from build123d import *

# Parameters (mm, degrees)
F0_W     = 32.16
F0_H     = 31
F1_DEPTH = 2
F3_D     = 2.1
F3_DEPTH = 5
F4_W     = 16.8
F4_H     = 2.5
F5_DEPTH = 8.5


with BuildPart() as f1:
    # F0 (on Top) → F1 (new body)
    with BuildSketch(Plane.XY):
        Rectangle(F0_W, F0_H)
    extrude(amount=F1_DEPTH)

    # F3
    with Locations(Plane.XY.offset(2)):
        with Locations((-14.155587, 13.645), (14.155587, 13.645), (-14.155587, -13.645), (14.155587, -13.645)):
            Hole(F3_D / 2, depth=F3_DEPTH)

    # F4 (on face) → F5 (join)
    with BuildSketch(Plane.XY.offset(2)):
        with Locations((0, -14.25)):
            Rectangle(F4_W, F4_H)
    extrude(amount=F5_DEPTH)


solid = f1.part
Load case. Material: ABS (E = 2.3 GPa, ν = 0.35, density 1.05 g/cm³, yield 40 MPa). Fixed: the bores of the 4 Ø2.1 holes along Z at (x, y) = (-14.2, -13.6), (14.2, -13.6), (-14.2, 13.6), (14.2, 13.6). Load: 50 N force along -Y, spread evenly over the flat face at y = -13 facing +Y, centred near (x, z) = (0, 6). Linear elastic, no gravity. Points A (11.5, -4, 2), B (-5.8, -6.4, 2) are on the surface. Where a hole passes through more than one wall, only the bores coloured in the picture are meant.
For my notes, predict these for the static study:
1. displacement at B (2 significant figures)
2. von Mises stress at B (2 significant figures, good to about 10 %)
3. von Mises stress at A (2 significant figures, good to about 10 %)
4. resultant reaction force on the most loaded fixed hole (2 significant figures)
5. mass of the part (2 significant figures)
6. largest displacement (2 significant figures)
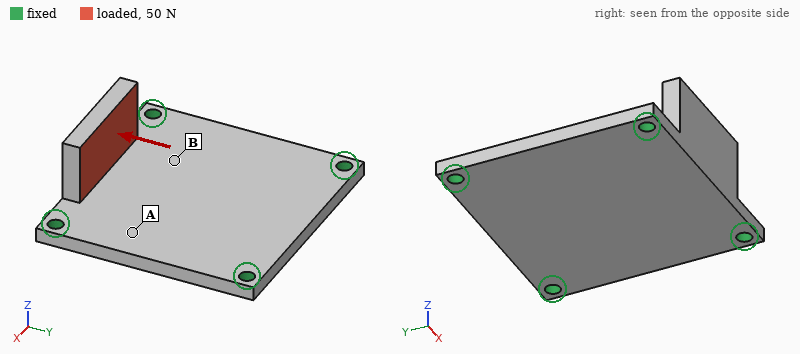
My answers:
0.089 mm
6.0 MPa
2.9 MPa
17 N
2.4 g
0.47 mm
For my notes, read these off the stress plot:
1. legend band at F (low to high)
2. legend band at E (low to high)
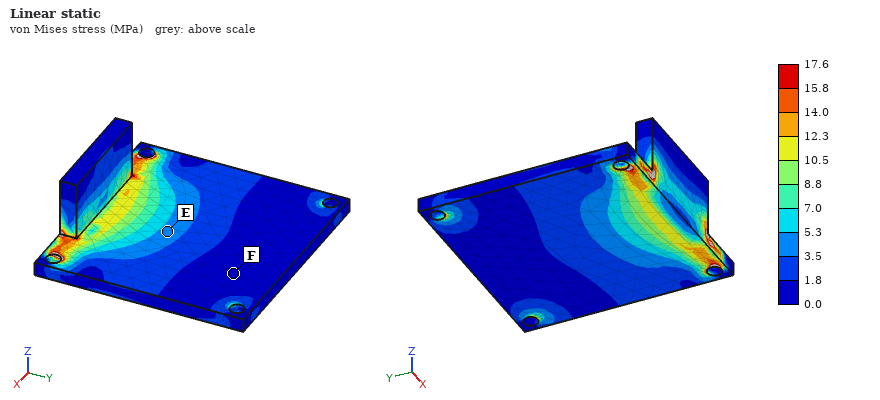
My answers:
0.0 to 1.8 MPa
3.5 to 5.3 MPa
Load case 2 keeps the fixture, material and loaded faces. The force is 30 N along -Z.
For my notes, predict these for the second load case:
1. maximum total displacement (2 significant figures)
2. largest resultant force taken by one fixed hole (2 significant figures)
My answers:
62 µm
16 N
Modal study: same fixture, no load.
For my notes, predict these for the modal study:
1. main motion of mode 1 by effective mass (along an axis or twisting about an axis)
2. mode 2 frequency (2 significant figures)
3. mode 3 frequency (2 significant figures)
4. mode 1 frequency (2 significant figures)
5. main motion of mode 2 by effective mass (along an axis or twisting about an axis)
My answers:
along Z
3500 Hz
4400 Hz
2500 Hz
along Z
